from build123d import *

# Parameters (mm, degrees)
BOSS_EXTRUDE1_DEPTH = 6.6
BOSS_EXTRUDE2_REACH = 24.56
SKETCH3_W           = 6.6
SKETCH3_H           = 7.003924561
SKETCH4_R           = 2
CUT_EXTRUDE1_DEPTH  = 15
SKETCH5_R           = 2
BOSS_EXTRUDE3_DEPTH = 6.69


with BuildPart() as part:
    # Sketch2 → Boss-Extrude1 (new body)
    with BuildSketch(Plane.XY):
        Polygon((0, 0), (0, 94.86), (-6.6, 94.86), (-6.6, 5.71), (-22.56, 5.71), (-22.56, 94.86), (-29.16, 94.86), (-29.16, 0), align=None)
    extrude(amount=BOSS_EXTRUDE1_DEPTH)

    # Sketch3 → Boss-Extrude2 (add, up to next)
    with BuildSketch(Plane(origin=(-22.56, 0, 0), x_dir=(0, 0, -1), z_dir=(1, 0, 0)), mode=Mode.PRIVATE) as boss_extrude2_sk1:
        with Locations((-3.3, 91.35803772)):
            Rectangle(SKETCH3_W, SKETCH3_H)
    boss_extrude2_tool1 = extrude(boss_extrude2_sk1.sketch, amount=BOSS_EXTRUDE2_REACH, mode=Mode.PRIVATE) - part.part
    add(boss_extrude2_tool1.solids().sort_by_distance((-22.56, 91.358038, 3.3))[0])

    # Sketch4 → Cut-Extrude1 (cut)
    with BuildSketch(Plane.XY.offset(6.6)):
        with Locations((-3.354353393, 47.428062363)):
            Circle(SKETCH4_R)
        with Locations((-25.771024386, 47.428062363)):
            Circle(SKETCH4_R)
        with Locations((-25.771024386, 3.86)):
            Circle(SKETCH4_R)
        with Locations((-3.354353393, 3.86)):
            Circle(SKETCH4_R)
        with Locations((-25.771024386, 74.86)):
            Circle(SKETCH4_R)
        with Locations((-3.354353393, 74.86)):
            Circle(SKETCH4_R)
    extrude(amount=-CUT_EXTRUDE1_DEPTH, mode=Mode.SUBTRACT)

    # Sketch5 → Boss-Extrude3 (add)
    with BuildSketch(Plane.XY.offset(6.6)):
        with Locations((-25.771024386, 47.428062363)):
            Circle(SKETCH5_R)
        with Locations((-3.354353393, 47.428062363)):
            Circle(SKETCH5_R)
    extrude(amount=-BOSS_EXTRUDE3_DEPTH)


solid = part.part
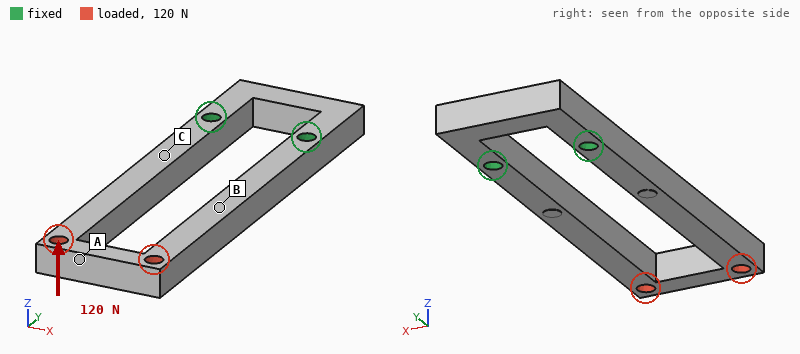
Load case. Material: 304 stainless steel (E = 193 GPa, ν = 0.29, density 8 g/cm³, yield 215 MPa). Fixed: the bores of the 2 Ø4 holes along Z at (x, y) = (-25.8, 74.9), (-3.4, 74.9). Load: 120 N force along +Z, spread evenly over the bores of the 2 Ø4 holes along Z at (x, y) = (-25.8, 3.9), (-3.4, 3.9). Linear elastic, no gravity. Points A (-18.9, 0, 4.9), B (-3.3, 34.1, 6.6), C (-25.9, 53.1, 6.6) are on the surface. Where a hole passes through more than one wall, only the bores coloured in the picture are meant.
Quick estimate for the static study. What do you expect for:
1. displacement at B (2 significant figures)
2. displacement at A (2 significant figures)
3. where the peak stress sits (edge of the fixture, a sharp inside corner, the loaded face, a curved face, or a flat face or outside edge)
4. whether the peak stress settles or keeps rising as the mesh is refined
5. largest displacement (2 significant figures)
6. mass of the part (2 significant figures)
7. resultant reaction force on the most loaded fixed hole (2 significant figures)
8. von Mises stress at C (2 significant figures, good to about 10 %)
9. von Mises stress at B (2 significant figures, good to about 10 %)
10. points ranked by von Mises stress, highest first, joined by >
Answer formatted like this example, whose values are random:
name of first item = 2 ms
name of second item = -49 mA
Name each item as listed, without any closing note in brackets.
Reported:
displacement at B = 0.088 mm
displacement at A = 0.24 mm
where the peak stress sits = edge of the fixture
whether the peak stress settles or keeps rising as the mesh is refined = keeps rising
largest displacement = 0.24 mm
mass of the part = 74 g
resultant reaction force on the most loaded fixed hole = 60 N
von Mises stress at C = 62 MPa
von Mises stress at B = 38 MPa
points ranked by von Mises stress, highest first, joined by > = C > B > A
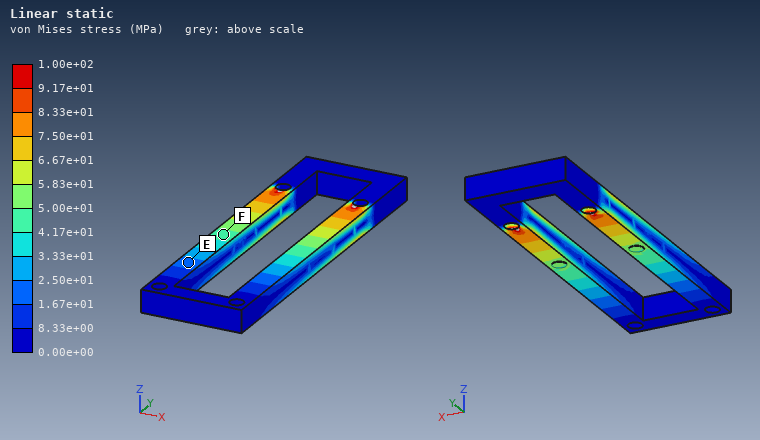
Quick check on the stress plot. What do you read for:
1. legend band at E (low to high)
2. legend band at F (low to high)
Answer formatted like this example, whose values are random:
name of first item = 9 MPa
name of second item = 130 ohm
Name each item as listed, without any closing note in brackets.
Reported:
legend band at E = 1.67e+01 to 2.50e+01 MPa
legend band at F = 4.17e+01 to 5.00e+01 MPa
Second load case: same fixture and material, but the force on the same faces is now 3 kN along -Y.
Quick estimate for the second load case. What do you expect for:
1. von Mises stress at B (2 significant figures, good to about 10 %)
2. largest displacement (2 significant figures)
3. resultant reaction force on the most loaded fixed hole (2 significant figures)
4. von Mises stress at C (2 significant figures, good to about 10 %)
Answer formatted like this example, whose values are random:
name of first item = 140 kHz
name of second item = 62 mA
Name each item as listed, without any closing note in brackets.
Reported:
von Mises stress at B = 34 MPa
largest displacement = 14 µm
resultant reaction force on the most loaded fixed hole = 1.5 kN
von Mises stress at C = 34 MPa
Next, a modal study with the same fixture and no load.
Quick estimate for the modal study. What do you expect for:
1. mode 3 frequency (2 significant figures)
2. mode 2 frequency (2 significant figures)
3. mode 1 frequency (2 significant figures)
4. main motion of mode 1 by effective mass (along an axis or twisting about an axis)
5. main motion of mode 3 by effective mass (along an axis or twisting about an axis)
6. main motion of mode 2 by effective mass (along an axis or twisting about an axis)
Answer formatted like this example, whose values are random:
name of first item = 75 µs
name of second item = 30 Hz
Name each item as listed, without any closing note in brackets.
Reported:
mode 3 frequency = 2600 Hz
mode 2 frequency = 1300 Hz
mode 1 frequency = 860 Hz
main motion of mode 1 by effective mass = along Z
main motion of mode 3 by effective mass = twisting about Y
main motion of mode 2 by effective mass = along X
